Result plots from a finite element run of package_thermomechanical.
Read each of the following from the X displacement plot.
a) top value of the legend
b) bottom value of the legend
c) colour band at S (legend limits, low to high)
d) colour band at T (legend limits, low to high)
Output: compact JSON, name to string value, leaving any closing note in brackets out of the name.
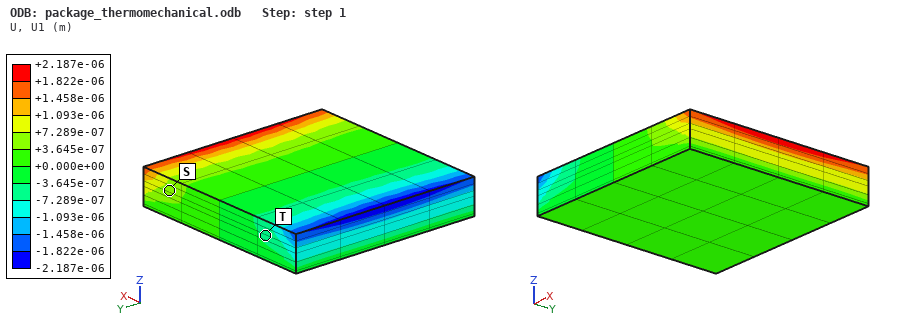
{"top value of the legend": "+2.187e-06 m", "bottom value of the legend": "-2.187e-06 m", "colour band at S": "+3.645e-07 to +7.289e-07 m", "colour band at T": "-7.289e-07 to -3.645e-07 m"}
